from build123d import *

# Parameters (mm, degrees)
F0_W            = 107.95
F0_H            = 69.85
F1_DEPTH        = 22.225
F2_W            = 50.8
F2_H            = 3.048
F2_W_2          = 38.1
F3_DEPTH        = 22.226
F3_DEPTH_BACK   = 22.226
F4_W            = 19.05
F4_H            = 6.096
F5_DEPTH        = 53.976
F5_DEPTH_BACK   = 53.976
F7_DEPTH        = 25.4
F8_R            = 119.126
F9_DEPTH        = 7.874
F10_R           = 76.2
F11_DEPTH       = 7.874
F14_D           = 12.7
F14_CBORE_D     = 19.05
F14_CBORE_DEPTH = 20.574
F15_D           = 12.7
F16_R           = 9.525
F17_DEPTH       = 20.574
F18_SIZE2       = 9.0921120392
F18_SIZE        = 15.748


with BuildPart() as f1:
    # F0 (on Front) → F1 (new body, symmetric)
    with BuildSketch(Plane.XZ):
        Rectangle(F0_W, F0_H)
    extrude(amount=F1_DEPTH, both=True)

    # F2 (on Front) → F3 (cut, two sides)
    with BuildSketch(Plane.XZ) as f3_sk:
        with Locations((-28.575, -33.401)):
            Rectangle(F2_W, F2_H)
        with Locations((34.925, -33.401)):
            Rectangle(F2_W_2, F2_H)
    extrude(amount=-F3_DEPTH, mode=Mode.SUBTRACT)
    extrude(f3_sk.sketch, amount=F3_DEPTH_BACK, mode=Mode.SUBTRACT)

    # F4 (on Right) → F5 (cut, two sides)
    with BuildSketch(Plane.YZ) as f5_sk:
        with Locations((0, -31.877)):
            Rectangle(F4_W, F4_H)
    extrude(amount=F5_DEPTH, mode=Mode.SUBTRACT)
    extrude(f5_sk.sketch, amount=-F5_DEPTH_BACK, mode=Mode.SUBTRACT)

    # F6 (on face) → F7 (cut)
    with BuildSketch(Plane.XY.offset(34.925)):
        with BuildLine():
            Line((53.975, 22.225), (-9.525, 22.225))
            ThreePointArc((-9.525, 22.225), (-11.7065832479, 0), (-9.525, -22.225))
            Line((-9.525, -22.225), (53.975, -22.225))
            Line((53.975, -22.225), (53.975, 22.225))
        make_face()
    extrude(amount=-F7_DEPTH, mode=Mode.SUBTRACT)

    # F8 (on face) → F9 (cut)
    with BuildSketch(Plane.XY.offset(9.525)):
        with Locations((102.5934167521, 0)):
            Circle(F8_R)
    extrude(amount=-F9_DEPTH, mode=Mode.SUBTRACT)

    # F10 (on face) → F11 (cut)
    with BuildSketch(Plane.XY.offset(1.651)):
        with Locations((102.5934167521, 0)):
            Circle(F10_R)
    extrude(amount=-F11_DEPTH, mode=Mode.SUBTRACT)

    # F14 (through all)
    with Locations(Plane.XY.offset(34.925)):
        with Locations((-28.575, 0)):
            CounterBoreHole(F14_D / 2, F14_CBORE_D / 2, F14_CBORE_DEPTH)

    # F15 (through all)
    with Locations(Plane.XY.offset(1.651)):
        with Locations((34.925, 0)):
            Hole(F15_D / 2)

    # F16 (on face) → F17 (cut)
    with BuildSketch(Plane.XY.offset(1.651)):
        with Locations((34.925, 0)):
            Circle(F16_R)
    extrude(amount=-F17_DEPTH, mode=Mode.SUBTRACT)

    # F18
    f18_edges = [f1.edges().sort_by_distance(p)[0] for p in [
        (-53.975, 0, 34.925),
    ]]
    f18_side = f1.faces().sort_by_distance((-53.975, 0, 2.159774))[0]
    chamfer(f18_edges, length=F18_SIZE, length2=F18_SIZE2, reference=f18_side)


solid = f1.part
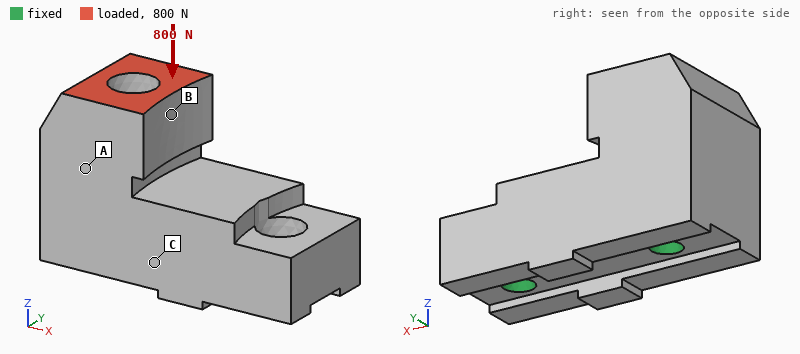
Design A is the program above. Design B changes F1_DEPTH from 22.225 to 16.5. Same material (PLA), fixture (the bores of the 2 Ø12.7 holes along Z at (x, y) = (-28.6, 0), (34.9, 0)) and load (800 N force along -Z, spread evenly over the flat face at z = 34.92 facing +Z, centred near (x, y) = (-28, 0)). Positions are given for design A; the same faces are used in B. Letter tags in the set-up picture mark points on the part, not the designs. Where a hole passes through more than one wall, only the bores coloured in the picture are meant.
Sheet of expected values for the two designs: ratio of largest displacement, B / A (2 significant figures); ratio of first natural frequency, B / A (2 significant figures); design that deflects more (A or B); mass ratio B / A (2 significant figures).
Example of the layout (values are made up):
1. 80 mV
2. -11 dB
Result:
1. 1.3
2. 1.2
3. B
4. 0.71
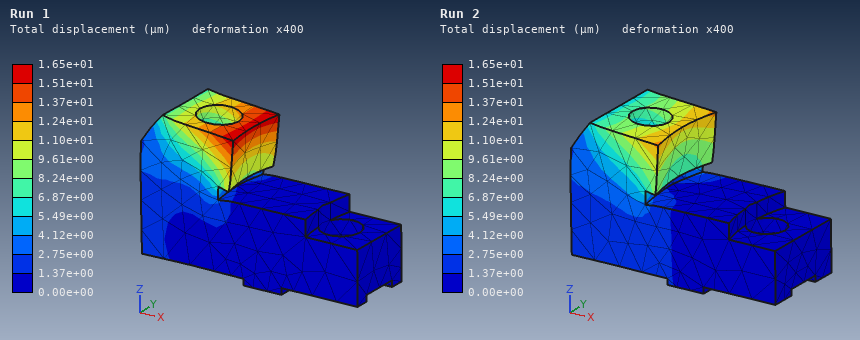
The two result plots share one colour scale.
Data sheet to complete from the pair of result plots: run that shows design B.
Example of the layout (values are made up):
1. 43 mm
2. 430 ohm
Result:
1. Run 1
